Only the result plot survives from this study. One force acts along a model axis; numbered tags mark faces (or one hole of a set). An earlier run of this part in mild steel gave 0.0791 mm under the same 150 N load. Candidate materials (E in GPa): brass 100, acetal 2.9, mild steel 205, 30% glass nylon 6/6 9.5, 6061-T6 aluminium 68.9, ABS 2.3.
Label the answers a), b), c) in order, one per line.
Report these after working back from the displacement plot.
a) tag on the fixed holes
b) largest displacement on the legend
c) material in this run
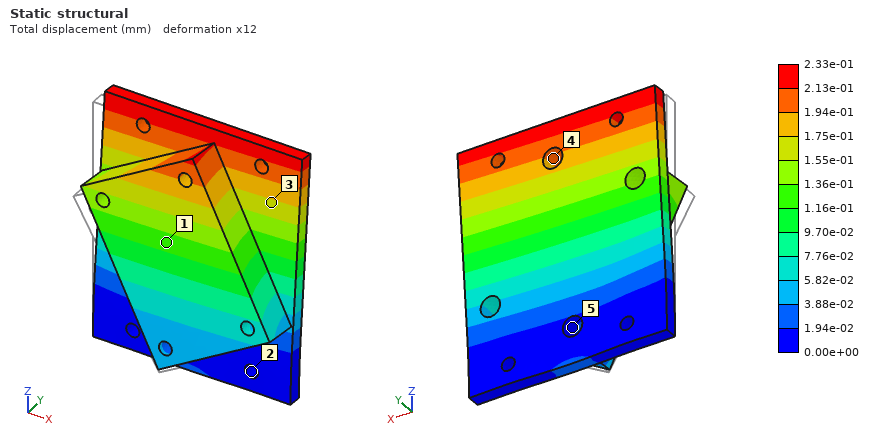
a) 2
b) 2.33e-01 mm
c) 6061-T6 aluminium
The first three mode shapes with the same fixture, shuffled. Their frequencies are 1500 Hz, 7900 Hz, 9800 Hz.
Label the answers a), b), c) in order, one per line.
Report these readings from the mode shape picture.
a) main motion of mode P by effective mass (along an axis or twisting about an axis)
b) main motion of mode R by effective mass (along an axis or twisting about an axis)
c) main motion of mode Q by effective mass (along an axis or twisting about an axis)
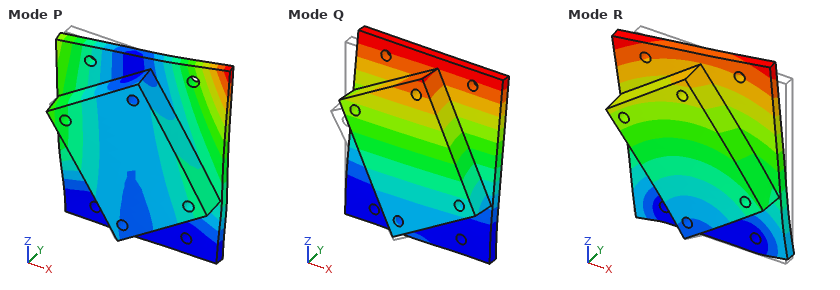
a) twisting about Z
b) along X
c) along Y
